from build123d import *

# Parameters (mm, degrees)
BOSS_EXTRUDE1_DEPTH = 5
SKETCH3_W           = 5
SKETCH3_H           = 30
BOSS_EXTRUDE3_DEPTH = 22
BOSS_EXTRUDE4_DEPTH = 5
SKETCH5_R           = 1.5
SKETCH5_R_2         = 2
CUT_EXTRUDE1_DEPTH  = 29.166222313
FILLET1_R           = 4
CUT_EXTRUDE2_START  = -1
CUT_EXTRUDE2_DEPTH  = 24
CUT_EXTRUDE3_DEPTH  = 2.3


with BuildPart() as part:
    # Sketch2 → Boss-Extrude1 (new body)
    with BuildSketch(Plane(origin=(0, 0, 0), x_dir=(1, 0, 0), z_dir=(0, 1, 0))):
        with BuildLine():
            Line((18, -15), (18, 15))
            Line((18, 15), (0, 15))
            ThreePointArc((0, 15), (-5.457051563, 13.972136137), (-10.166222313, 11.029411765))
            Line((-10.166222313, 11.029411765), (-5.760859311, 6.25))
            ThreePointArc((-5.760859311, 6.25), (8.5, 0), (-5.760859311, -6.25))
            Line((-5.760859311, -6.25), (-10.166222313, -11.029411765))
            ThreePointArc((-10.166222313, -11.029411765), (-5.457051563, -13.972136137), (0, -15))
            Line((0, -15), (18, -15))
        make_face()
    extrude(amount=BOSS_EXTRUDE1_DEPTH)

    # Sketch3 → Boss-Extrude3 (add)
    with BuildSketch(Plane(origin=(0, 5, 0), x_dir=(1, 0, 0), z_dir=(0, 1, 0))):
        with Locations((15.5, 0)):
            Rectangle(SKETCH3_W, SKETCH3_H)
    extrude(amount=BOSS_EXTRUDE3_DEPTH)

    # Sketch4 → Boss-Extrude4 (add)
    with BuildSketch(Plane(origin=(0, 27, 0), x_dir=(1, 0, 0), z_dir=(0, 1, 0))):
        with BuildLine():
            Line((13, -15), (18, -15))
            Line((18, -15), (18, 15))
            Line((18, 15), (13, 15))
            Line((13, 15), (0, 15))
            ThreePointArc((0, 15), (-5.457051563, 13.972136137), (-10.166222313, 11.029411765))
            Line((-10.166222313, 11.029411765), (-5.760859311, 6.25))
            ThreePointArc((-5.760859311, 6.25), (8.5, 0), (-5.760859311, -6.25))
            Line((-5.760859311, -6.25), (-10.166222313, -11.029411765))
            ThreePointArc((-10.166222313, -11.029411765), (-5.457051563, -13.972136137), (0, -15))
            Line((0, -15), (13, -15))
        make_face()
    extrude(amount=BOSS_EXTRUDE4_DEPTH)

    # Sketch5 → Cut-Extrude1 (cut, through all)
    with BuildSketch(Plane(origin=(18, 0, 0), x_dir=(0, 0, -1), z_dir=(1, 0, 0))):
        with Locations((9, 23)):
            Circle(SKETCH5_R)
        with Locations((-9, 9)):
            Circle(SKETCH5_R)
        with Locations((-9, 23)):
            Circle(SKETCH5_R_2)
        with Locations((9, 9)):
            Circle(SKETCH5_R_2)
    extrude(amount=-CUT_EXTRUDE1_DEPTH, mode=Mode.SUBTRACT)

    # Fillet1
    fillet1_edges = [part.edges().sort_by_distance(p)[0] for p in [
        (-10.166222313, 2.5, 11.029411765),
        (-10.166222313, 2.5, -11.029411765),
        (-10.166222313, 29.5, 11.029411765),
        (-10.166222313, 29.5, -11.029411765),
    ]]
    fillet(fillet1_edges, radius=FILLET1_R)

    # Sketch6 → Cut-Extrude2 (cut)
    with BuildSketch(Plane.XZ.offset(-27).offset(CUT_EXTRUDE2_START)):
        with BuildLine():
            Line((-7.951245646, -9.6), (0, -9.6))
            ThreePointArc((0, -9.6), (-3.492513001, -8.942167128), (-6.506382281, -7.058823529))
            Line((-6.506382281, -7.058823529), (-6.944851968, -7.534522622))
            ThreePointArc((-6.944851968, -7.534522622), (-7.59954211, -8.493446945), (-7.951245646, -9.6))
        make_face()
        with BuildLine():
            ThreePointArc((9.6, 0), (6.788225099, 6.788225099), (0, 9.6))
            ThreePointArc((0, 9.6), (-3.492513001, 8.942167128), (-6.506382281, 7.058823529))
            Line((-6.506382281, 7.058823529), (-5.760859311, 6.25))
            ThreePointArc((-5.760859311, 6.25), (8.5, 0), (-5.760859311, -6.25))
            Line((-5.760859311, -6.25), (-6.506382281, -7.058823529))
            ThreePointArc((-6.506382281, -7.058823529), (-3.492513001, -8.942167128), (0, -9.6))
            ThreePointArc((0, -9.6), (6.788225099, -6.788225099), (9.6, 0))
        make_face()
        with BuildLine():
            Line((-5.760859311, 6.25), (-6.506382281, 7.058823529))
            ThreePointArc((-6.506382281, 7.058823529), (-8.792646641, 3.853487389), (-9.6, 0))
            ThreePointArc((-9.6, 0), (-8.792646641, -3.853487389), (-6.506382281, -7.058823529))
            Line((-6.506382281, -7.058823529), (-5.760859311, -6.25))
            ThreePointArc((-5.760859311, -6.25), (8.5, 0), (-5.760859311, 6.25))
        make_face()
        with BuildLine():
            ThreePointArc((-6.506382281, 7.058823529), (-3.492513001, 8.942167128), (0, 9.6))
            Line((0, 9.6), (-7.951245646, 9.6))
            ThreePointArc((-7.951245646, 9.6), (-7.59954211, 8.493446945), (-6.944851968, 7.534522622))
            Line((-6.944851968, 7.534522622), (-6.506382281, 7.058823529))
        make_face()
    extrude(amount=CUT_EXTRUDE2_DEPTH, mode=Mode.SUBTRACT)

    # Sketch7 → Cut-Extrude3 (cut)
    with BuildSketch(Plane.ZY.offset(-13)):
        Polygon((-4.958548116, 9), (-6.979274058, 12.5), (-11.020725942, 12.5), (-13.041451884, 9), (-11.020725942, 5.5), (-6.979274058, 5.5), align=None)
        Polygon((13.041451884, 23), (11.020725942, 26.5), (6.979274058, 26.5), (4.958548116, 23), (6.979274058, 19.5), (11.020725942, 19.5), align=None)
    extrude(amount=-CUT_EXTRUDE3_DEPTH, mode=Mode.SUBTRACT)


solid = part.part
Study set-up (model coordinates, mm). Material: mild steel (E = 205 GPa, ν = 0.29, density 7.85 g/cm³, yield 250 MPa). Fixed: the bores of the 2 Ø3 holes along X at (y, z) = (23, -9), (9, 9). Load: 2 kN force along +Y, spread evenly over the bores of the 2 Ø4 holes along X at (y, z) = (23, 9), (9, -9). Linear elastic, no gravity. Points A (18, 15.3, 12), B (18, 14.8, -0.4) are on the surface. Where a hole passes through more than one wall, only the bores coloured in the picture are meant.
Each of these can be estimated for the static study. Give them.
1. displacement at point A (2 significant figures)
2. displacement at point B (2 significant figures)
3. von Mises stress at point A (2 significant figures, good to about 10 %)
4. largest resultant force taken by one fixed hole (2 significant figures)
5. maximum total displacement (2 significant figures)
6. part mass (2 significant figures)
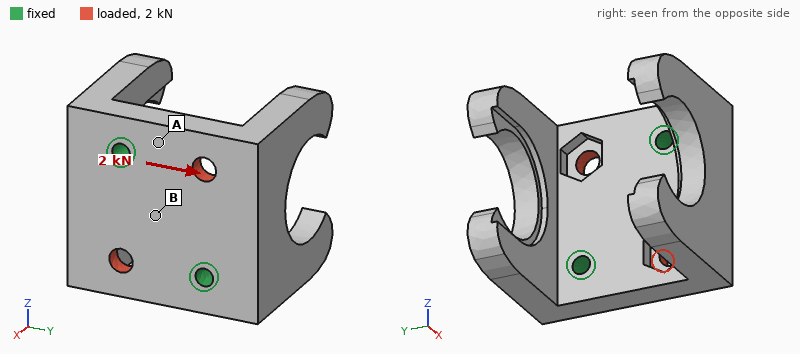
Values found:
0.97 µm
1.1 µm
28 MPa
1.0 kN
4.6 µm
64 g
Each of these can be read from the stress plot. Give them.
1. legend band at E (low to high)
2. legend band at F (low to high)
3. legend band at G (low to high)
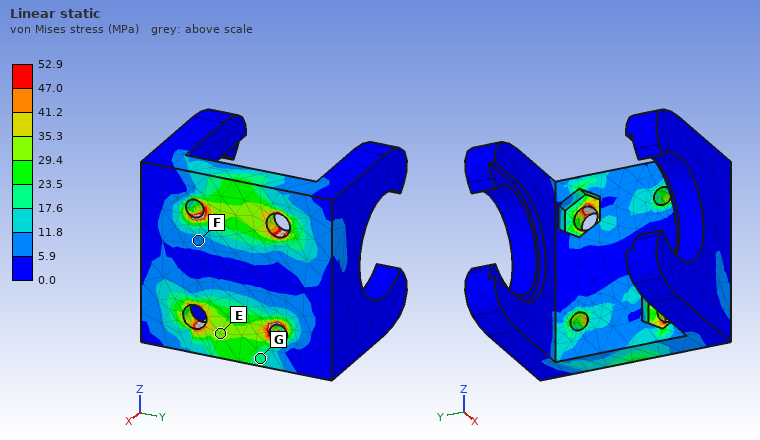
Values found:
29.4 to 35.3 MPa
5.9 to 11.8 MPa
17.6 to 23.5 MPa
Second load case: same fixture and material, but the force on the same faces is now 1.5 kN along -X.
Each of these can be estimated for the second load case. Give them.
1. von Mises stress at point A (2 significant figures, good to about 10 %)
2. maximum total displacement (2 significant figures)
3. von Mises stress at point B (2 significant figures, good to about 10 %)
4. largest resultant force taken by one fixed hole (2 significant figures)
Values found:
33 MPa
19 µm
53 MPa
750 N
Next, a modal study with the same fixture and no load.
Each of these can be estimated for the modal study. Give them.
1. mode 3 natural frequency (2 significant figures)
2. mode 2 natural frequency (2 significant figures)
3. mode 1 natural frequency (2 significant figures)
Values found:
7800 Hz
5800 Hz
5200 Hz
